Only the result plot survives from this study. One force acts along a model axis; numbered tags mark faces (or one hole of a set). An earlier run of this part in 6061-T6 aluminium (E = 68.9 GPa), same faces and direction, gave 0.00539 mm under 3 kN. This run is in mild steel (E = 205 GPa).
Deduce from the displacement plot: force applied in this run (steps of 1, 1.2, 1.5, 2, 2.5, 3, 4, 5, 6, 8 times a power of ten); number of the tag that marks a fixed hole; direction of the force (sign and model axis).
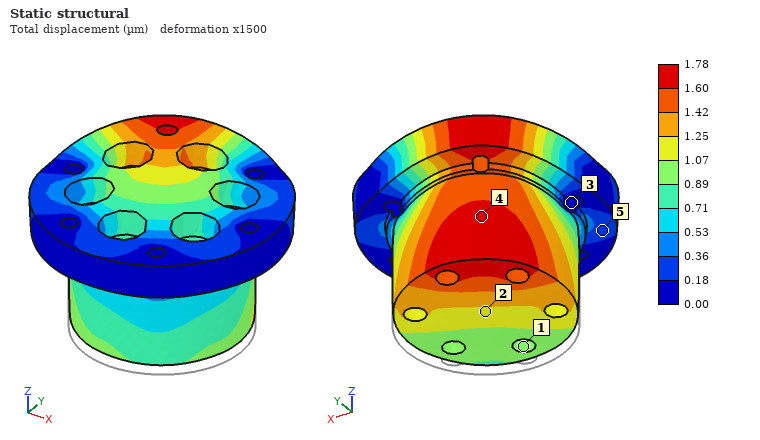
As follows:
3 kN
3
+Z
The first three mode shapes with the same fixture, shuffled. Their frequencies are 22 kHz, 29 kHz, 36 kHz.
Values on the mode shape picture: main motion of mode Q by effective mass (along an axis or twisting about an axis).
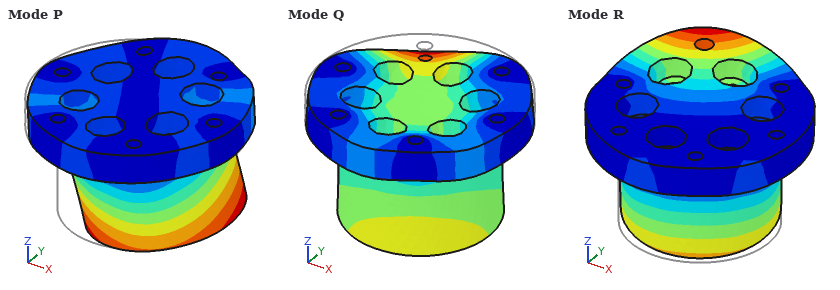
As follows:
along Z
